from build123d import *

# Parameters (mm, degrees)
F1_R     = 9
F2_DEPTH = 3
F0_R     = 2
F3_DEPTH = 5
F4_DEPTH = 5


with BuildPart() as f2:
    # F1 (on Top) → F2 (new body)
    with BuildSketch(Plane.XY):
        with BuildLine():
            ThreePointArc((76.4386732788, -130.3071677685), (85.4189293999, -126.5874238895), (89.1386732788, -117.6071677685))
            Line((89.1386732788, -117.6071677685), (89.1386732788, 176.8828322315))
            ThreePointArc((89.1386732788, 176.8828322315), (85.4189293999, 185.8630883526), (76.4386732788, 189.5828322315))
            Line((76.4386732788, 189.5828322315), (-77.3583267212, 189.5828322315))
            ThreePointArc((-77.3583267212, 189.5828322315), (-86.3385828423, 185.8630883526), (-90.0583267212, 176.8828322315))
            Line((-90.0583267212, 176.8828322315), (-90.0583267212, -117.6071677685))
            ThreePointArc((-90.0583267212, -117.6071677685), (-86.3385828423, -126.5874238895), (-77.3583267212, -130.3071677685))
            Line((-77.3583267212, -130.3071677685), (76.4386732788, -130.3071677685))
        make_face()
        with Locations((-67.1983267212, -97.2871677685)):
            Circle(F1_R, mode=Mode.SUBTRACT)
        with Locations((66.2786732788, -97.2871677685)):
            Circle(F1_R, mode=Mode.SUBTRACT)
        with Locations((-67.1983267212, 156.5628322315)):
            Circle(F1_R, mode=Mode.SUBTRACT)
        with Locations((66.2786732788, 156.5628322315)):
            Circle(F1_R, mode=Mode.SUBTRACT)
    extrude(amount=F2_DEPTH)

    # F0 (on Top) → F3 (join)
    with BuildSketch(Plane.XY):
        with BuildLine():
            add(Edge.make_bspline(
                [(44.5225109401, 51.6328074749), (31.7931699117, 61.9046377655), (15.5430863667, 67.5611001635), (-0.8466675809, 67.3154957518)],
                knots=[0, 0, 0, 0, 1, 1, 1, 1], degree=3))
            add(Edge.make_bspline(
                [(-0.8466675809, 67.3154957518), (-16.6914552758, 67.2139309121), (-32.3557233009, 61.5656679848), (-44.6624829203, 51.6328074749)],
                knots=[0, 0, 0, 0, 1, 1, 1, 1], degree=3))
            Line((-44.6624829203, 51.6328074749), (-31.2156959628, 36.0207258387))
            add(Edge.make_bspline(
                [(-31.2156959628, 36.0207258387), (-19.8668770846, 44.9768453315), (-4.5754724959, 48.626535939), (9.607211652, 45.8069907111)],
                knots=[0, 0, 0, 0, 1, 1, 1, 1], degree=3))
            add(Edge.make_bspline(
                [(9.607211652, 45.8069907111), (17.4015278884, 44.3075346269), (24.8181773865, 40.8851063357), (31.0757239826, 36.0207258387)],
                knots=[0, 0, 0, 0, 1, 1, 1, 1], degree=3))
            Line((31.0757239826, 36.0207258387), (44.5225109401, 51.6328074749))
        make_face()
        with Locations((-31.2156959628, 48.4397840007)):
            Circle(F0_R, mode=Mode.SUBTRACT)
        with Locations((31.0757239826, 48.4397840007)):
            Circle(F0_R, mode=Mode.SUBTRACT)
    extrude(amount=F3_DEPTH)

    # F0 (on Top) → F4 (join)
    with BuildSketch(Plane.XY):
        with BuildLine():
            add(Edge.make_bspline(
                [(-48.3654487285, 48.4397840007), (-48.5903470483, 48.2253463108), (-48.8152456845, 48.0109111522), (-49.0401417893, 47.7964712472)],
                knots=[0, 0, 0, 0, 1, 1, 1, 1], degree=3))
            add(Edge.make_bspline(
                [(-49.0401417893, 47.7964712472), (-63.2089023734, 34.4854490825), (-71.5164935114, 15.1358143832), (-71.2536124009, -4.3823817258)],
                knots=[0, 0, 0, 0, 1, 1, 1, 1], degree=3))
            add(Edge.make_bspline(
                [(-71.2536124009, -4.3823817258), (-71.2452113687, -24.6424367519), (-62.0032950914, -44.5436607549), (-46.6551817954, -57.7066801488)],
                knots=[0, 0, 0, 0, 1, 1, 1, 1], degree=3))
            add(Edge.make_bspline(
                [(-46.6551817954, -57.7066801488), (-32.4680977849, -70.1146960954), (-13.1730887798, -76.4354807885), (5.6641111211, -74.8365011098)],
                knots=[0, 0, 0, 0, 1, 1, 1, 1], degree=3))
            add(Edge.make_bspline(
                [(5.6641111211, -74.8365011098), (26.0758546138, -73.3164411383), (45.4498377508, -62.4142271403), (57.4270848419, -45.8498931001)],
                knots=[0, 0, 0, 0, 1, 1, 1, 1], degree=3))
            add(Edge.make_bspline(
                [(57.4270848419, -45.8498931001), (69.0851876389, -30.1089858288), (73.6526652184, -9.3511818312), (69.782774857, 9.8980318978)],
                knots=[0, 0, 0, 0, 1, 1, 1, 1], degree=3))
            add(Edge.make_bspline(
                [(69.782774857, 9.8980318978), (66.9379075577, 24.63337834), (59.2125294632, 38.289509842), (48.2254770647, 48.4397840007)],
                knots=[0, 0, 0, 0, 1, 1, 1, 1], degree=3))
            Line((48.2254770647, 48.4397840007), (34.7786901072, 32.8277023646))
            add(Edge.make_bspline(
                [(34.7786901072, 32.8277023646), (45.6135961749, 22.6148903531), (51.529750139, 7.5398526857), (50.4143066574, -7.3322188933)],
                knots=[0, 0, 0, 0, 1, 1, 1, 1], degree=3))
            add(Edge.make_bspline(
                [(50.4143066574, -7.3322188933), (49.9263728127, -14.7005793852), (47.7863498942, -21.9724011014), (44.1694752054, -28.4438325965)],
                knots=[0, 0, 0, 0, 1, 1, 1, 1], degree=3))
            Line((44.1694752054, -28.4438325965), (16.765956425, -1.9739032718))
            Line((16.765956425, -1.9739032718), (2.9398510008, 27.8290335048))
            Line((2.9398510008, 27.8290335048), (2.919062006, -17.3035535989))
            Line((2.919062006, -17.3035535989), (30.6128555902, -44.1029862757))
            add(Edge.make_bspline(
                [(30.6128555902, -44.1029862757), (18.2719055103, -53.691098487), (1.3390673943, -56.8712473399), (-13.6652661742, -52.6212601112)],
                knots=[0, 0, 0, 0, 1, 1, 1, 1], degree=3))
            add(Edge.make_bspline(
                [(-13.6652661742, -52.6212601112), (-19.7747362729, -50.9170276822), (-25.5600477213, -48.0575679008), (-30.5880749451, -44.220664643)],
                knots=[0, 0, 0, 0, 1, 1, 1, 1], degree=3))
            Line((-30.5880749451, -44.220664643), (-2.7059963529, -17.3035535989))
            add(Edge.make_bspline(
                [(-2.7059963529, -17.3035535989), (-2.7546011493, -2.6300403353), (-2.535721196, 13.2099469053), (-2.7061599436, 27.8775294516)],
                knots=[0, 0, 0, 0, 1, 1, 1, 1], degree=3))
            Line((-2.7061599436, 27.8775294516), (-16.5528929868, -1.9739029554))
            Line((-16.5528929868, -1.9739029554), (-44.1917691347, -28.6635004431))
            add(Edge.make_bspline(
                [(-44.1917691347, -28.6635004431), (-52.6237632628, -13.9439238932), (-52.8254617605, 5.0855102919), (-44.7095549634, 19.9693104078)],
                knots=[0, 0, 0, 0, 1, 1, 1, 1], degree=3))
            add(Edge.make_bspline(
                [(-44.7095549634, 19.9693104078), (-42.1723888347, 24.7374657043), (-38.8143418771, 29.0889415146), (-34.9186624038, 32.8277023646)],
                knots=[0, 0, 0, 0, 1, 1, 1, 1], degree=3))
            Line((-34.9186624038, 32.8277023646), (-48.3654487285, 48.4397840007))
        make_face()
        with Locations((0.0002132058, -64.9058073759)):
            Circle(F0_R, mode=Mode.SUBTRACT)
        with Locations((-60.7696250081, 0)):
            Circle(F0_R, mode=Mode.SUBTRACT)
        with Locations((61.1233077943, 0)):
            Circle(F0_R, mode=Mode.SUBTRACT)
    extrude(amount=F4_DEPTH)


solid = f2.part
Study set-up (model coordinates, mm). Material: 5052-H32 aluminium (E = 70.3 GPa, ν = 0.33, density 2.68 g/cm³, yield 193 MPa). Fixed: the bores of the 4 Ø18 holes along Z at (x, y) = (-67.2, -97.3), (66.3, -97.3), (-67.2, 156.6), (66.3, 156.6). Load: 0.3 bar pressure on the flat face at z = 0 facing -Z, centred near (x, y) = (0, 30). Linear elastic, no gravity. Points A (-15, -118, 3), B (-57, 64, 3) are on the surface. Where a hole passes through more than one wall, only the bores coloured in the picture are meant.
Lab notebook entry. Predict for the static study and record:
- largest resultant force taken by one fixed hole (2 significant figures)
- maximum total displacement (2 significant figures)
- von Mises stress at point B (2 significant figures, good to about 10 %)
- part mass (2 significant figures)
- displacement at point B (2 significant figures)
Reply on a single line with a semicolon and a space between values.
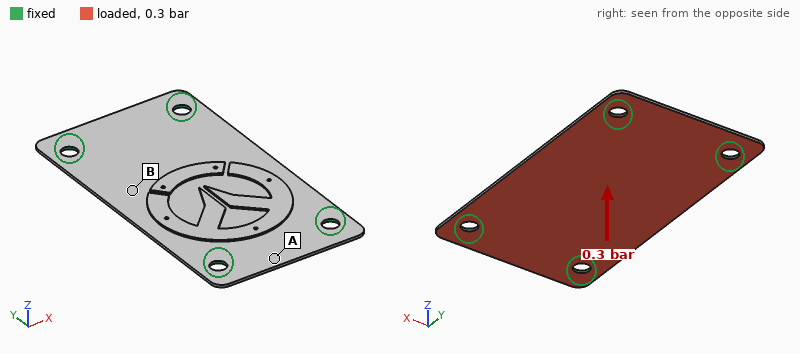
650 N; 1.5 mm; 44 MPa; 500 g; 1.4 mm
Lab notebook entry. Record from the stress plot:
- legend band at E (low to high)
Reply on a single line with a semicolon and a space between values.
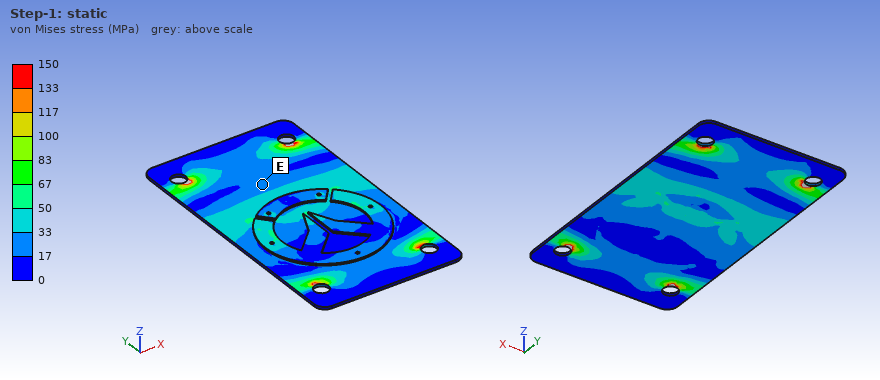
17 to 33 MPa
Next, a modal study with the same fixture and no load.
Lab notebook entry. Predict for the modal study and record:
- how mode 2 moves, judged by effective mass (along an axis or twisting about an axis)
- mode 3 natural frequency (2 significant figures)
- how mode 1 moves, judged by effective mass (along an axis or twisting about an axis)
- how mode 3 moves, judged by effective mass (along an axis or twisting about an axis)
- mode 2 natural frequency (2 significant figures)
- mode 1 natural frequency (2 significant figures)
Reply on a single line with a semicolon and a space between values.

twisting about Y; 740 Hz; along Z; twisting about X; 410 Hz; 260 Hz
